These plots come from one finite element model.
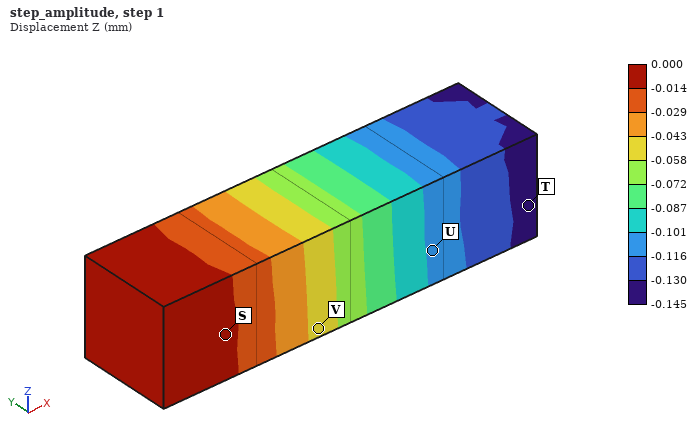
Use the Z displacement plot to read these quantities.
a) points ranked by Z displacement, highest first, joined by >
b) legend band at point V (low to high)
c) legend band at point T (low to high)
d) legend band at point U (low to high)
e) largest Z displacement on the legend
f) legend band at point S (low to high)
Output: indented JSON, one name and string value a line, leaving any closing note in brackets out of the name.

{
  "points ranked by Z displacement, highest first, joined by >": "S > V > U > T",
  "legend band at point V": "-0.058 to -0.043 mm",
  "legend band at point T": "-0.145 to -0.130 mm",
  "legend band at point U": "-0.116 to -0.101 mm",
  "largest Z displacement on the legend": "0.000 mm",
  "legend band at point S": "-0.014 to 0.000 mm"
}
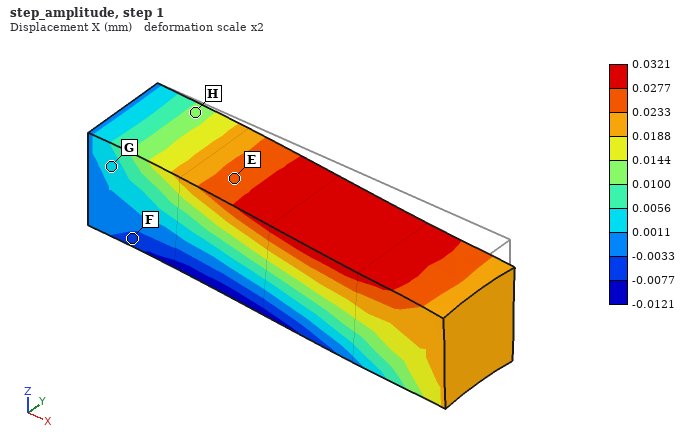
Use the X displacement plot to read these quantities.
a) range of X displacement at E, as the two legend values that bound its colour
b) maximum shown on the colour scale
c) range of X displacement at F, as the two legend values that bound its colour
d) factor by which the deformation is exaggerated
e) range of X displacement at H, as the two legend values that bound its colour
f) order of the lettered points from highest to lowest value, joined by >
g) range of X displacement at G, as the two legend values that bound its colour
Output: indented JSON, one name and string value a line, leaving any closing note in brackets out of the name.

{
  "range of X displacement at E, as the two legend values that bound its colour": "0.0233 to 0.0277 mm",
  "maximum shown on the colour scale": "0.0321 mm",
  "range of X displacement at F, as the two legend values that bound its colour": "-0.0077 to -0.0033 mm",
  "factor by which the deformation is exaggerated": "2",
  "range of X displacement at H, as the two legend values that bound its colour": "0.0100 to 0.0144 mm",
  "order of the lettered points from highest to lowest value, joined by >": "E > H > G > F",
  "range of X displacement at G, as the two legend values that bound its colour": "0.0011 to 0.0056 mm"
}
